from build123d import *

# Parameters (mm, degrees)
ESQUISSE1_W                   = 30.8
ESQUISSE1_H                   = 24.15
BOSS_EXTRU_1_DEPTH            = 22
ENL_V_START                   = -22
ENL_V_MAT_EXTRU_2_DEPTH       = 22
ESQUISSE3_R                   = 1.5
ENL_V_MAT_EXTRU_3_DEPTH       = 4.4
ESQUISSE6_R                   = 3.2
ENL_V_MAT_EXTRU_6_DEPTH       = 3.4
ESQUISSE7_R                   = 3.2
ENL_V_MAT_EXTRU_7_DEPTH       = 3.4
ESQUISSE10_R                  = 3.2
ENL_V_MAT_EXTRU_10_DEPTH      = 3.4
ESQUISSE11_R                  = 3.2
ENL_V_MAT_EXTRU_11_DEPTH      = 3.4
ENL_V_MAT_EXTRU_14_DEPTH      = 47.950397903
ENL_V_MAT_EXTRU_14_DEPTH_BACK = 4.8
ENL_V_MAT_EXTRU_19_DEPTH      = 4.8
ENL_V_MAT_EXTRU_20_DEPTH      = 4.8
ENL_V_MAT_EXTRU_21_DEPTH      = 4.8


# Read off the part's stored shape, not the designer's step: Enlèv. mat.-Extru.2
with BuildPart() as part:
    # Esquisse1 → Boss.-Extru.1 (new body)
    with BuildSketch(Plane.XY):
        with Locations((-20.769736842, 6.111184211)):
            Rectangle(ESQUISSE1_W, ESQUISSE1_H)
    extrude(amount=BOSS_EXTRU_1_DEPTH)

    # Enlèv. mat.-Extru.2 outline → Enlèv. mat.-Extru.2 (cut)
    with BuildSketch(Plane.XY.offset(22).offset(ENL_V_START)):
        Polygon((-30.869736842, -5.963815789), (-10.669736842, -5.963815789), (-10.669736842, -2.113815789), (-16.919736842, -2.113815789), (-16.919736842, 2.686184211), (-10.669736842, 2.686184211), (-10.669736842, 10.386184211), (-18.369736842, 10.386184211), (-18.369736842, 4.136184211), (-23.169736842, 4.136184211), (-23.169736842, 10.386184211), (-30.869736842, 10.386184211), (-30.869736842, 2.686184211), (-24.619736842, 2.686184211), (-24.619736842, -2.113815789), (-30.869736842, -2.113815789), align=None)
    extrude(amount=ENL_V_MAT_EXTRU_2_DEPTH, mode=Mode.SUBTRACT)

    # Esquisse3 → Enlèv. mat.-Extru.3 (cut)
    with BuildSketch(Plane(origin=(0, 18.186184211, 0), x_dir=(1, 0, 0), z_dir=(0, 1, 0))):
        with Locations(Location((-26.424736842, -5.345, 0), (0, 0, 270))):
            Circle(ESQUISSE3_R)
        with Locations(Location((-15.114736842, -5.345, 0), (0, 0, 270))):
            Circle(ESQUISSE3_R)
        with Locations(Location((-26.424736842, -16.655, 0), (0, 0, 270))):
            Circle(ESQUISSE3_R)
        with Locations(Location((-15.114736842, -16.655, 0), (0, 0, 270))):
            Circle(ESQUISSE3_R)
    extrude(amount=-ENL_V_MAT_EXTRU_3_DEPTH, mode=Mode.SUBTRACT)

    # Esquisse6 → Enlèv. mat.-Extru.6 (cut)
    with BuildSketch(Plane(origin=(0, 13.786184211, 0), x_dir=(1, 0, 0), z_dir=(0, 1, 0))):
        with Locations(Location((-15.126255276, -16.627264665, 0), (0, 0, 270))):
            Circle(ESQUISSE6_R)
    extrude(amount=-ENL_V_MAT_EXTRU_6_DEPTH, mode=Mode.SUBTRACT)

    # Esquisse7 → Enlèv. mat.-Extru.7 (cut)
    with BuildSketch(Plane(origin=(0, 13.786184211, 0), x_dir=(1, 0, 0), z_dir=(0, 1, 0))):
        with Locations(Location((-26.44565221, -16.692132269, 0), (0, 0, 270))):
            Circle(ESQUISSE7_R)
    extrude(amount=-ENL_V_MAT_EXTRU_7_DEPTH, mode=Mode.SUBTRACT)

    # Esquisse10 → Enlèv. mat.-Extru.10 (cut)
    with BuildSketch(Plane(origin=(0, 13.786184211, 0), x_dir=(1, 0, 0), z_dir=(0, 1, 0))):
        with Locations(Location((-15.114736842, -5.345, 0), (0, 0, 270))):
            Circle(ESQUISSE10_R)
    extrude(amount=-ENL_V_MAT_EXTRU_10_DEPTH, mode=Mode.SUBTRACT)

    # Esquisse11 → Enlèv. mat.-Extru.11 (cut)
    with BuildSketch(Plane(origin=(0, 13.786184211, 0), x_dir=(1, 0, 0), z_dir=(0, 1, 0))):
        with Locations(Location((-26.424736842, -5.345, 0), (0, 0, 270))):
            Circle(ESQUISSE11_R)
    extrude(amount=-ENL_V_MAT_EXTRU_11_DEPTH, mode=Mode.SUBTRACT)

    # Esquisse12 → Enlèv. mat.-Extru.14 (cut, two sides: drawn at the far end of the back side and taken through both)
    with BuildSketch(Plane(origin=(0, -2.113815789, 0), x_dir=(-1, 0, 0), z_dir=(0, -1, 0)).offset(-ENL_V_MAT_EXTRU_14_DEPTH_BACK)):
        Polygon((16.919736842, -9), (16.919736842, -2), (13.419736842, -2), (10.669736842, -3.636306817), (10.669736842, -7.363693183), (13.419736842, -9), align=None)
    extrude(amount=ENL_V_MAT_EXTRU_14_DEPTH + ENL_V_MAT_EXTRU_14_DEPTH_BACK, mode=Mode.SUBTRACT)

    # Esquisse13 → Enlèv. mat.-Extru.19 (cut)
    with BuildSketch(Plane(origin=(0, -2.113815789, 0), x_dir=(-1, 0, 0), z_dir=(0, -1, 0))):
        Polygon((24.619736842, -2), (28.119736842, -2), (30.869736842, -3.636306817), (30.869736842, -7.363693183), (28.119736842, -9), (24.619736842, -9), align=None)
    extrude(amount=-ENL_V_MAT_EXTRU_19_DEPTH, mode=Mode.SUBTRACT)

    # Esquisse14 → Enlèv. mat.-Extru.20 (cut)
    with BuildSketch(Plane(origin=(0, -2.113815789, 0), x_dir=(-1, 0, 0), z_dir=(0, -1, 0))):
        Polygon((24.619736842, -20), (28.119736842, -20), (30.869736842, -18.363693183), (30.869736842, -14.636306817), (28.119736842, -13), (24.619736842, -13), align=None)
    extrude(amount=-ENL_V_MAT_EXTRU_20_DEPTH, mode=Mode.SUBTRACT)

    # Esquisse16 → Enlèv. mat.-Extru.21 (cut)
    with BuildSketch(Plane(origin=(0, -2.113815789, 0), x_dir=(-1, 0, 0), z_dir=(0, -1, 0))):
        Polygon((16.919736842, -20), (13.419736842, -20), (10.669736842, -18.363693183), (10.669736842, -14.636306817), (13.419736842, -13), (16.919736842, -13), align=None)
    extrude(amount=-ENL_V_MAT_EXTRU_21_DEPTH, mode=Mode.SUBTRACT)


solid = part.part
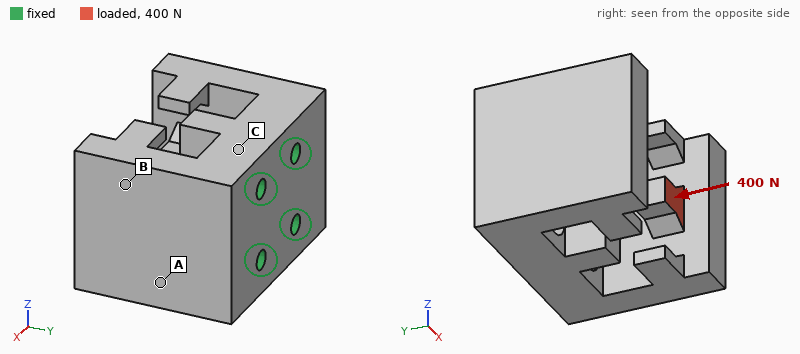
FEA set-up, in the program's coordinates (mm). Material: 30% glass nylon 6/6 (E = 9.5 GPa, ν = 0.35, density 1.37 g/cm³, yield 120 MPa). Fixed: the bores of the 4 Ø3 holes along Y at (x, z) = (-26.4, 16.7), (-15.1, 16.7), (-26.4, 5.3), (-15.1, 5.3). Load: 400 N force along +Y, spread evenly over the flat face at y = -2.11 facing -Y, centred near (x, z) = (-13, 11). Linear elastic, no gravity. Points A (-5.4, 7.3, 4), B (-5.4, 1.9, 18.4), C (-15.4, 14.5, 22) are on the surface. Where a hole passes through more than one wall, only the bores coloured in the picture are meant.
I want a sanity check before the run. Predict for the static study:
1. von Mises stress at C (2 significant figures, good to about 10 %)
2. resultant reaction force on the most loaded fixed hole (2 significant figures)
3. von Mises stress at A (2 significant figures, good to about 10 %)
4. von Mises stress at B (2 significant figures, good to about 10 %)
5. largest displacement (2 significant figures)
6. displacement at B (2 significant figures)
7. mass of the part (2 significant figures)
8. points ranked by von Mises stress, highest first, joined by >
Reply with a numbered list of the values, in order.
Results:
1. 3.9 MPa
2. 200 N
3. 16 MPa
4. 11 MPa
5. 0.19 mm
6. 0.047 mm
7. 13 g
8. A > B > C
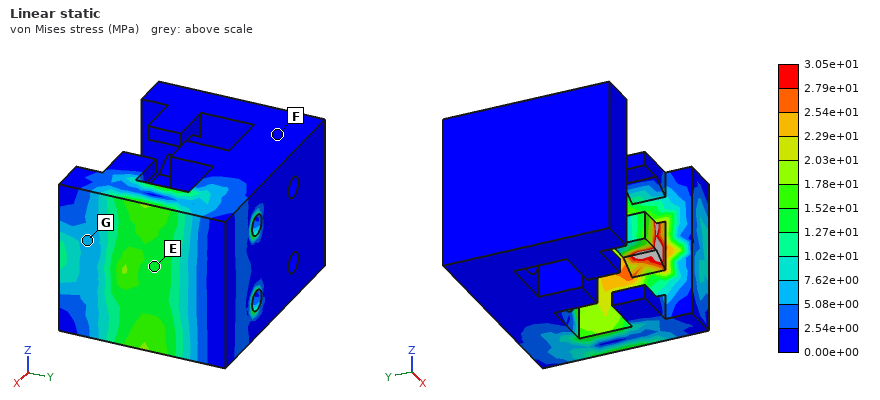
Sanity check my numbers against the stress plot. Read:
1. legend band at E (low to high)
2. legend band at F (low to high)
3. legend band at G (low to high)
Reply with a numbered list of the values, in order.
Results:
1. 1.27e+01 to 1.52e+01 MPa
2. 0.00e+00 to 2.54e+00 MPa
3. 5.08e+00 to 7.62e+00 MPa
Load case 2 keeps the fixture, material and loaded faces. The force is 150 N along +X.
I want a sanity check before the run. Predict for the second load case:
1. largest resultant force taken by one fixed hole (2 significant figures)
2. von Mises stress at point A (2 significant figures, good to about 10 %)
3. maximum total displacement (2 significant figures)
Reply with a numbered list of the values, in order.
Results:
1. 100 N
2. 13 MPa
3. 0.17 mm
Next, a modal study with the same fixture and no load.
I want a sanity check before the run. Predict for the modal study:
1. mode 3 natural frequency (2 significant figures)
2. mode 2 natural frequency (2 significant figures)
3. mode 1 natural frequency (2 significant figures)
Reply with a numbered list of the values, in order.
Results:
1. 6400 Hz
2. 4000 Hz
3. 3900 Hz
